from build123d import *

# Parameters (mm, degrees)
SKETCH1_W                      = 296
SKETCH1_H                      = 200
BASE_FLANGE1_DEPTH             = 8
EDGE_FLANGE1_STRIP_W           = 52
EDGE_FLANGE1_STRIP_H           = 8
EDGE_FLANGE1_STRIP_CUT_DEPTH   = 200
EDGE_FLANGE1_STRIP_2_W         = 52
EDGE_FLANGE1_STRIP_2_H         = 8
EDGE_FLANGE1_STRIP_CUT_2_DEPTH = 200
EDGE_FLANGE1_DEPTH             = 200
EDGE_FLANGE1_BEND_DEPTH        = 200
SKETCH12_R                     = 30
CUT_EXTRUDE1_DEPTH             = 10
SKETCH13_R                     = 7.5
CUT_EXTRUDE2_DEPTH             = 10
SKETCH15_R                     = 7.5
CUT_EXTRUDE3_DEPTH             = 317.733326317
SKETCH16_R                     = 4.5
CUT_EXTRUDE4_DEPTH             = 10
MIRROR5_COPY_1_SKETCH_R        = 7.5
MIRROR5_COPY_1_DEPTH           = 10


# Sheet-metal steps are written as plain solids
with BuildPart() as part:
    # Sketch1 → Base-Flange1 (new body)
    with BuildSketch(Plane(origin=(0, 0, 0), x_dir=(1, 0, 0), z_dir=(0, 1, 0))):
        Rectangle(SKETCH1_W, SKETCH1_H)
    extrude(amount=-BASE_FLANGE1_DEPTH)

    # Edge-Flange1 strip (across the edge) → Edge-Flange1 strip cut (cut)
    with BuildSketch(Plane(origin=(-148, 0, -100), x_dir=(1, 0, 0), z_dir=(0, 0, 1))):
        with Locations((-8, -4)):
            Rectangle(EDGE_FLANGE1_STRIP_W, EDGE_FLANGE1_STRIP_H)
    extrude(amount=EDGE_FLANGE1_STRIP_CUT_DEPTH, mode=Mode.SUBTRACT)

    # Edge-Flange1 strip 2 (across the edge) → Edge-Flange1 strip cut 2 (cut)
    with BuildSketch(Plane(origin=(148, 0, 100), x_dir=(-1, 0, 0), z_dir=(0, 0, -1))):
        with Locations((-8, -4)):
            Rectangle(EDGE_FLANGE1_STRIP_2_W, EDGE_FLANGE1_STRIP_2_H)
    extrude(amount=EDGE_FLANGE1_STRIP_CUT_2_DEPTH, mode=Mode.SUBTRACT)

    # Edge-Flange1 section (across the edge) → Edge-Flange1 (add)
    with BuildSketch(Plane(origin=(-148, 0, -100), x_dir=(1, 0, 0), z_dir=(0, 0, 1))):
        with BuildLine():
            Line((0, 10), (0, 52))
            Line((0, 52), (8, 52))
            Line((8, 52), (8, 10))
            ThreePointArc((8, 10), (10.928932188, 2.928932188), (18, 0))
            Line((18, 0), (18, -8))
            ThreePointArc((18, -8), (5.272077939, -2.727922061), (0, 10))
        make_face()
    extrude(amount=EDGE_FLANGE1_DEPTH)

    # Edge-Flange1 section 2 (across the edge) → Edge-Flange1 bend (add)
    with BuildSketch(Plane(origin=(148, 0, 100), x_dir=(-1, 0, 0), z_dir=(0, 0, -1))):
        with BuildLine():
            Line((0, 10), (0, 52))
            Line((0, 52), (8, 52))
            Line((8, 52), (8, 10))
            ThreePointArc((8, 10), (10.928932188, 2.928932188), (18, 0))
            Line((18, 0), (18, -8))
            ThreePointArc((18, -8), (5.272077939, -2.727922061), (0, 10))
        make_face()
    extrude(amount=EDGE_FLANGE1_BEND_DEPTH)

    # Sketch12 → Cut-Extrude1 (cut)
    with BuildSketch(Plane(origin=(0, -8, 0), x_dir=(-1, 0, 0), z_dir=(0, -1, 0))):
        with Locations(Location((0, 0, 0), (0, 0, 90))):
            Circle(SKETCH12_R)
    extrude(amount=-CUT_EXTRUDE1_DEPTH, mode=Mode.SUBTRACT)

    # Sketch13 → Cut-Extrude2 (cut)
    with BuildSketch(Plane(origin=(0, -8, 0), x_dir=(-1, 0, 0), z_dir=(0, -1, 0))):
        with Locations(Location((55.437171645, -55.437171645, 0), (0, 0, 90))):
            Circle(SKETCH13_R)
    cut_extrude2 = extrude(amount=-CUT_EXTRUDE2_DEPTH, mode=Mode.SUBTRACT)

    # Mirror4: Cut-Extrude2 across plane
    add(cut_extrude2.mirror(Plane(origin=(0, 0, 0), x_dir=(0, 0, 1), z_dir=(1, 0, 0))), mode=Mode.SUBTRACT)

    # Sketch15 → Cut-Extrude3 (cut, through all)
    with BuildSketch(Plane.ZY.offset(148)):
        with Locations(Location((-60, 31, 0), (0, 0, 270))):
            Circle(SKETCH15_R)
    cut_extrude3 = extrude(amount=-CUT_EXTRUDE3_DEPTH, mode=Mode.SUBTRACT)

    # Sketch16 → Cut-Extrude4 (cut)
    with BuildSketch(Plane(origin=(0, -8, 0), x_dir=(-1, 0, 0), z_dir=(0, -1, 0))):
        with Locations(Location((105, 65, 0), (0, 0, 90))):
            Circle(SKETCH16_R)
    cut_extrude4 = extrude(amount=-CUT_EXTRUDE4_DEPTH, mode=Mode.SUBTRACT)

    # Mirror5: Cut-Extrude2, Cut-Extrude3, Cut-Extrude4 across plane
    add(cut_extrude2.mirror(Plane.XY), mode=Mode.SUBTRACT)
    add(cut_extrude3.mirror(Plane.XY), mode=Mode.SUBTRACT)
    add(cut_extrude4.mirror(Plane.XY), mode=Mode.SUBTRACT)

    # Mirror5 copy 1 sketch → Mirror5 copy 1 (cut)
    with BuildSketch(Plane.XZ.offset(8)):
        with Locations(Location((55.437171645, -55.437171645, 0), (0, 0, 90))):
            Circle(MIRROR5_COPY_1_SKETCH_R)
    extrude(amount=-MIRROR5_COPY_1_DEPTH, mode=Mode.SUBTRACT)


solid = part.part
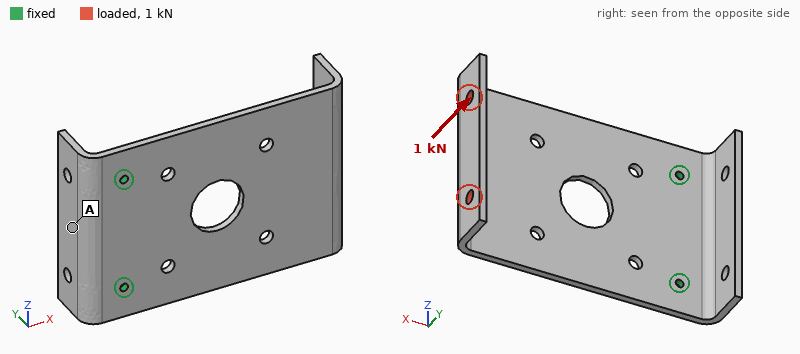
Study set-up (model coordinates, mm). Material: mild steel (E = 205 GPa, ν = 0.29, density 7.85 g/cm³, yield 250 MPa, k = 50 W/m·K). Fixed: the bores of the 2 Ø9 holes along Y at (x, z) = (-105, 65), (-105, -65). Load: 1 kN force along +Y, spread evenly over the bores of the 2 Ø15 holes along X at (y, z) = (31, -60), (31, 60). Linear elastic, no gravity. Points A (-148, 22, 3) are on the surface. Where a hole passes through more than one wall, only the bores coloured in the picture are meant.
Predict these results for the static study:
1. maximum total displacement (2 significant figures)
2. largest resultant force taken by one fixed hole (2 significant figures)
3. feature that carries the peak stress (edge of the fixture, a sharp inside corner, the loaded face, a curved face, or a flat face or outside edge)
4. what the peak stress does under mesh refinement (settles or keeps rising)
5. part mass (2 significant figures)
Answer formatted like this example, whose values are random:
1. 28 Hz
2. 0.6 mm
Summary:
1. 3.9 mm
2. 500 N
3. edge of the fixture
4. keeps rising
5. 4.6 kg
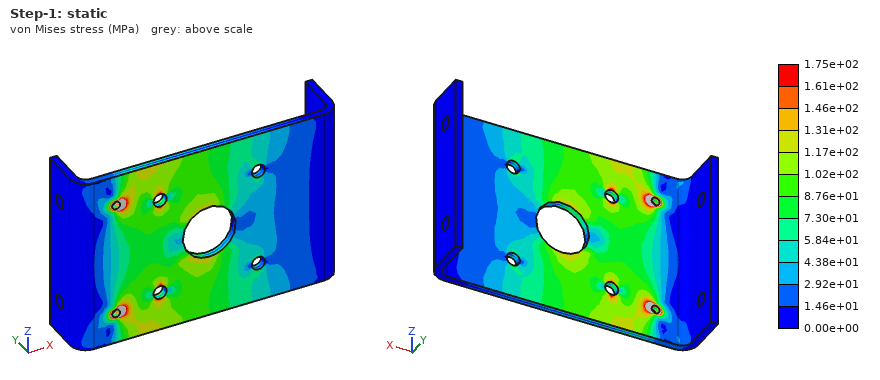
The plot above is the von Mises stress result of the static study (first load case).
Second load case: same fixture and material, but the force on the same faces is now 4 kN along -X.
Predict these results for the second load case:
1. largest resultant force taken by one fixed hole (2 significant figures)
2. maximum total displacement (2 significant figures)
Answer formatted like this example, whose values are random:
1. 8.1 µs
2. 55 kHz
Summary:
1. 2.0 kN
2. 3.4 mm
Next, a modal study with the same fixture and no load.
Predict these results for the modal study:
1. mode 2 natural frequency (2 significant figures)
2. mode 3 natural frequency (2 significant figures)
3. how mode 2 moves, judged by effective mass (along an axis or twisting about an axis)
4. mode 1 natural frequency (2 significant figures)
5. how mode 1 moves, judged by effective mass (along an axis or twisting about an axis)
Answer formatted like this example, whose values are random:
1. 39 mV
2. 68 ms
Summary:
1. 230 Hz
2. 470 Hz
3. twisting about X
4. 72 Hz
5. along Y
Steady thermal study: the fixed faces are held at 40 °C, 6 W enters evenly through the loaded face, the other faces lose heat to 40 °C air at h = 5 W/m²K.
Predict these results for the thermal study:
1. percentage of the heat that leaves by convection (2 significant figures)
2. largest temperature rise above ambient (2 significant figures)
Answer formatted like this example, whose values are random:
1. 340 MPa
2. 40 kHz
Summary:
1. 67 %
2. 14 K
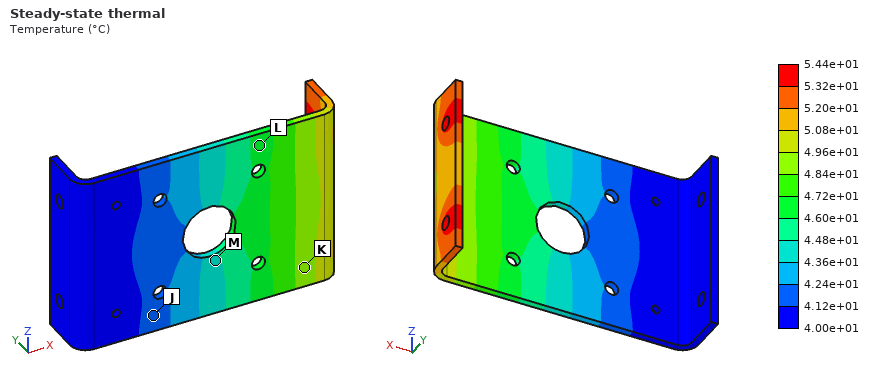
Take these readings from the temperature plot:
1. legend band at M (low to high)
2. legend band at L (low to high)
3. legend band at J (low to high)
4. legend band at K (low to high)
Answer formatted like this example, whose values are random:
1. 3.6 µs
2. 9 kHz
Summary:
1. 4.36e+01 to 4.48e+01 °C
2. 4.60e+01 to 4.72e+01 °C
3. 4.12e+01 to 4.24e+01 °C
4. 4.84e+01 to 4.96e+01 °C
